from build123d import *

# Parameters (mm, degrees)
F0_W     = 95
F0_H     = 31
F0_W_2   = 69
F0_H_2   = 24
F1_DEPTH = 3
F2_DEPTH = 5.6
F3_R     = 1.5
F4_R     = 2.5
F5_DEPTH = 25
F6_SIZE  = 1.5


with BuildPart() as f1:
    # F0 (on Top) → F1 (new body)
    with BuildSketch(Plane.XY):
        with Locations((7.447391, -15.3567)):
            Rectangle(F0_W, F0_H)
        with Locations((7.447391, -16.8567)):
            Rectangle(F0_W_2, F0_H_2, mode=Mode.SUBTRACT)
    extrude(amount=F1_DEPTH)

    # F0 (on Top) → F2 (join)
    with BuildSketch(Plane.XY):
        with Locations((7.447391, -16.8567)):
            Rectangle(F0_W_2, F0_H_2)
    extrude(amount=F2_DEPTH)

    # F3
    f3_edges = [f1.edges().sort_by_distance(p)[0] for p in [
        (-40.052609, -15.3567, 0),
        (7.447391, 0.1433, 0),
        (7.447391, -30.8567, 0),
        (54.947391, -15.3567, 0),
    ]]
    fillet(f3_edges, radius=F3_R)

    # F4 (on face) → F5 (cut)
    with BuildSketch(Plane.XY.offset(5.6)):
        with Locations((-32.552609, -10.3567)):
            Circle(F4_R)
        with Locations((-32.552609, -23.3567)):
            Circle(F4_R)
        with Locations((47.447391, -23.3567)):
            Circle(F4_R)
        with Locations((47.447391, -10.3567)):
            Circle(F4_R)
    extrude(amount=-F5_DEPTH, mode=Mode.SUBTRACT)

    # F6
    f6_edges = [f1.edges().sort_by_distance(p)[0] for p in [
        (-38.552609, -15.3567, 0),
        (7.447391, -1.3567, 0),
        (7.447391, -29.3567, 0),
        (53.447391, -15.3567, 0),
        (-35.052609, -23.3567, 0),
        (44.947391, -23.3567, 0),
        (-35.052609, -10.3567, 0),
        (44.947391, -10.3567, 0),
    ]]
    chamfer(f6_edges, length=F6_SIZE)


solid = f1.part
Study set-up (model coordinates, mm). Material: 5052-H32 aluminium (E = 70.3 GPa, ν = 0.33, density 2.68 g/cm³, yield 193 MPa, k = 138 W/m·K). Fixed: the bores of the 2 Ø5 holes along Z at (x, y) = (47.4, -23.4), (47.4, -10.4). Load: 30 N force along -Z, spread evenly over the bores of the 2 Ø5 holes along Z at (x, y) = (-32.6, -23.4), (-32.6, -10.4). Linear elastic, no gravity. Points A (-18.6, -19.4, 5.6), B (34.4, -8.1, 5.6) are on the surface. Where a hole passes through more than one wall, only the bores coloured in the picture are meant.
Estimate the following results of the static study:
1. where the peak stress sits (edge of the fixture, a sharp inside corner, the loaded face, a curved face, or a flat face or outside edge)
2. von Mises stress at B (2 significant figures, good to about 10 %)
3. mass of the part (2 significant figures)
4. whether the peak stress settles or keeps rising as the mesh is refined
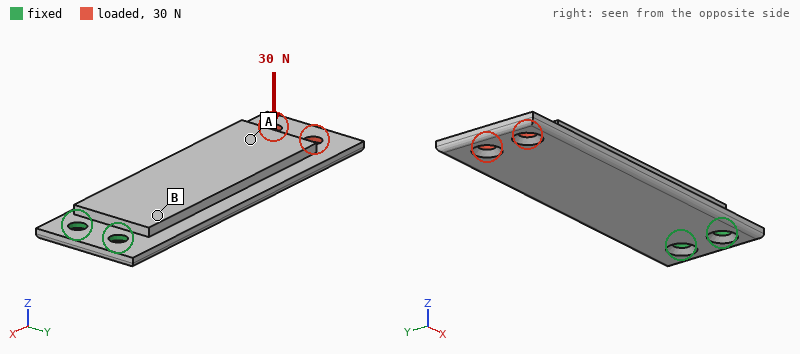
edge of the fixture
16 MPa
34 g
keeps rising
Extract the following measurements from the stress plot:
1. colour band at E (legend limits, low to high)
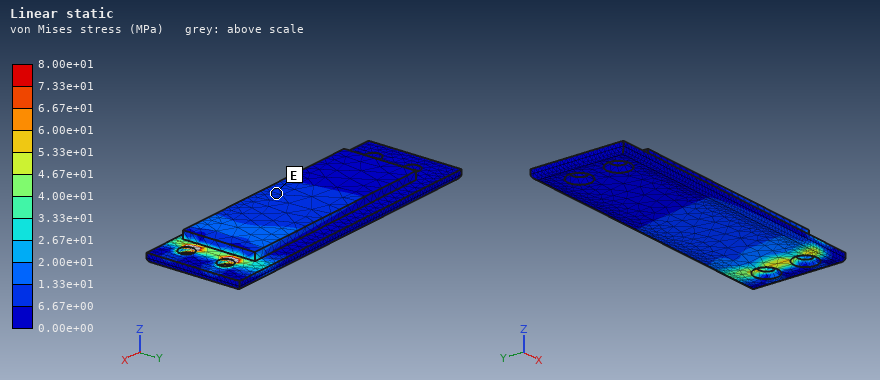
6.67e+00 to 1.33e+01 MPa
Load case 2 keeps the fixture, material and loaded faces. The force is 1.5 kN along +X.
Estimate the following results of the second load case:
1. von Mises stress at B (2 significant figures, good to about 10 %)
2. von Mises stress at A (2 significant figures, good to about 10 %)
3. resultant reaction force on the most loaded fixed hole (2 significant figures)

5.0 MPa
5.6 MPa
760 N
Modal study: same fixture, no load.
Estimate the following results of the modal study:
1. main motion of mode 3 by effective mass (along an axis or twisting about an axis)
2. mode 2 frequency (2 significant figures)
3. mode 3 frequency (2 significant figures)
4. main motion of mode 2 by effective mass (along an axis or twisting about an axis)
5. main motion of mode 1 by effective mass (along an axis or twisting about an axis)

twisting about X
2500 Hz
3100 Hz
along Y
along Z
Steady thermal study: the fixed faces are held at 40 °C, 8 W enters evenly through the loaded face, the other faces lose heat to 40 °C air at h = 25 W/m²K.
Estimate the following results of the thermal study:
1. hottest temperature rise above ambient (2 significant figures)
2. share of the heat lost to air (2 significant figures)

30 K
28 %
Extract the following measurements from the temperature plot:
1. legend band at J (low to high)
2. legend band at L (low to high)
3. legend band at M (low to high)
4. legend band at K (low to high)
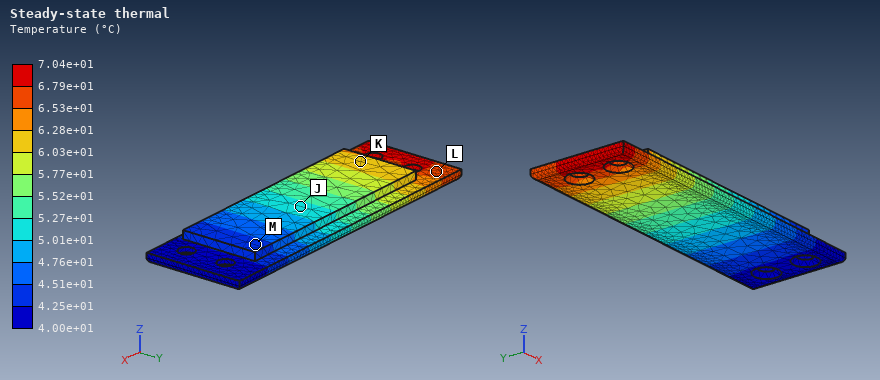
5.01e+01 to 5.27e+01 °C
6.53e+01 to 6.79e+01 °C
4.25e+01 to 4.51e+01 °C
6.03e+01 to 6.28e+01 °C
